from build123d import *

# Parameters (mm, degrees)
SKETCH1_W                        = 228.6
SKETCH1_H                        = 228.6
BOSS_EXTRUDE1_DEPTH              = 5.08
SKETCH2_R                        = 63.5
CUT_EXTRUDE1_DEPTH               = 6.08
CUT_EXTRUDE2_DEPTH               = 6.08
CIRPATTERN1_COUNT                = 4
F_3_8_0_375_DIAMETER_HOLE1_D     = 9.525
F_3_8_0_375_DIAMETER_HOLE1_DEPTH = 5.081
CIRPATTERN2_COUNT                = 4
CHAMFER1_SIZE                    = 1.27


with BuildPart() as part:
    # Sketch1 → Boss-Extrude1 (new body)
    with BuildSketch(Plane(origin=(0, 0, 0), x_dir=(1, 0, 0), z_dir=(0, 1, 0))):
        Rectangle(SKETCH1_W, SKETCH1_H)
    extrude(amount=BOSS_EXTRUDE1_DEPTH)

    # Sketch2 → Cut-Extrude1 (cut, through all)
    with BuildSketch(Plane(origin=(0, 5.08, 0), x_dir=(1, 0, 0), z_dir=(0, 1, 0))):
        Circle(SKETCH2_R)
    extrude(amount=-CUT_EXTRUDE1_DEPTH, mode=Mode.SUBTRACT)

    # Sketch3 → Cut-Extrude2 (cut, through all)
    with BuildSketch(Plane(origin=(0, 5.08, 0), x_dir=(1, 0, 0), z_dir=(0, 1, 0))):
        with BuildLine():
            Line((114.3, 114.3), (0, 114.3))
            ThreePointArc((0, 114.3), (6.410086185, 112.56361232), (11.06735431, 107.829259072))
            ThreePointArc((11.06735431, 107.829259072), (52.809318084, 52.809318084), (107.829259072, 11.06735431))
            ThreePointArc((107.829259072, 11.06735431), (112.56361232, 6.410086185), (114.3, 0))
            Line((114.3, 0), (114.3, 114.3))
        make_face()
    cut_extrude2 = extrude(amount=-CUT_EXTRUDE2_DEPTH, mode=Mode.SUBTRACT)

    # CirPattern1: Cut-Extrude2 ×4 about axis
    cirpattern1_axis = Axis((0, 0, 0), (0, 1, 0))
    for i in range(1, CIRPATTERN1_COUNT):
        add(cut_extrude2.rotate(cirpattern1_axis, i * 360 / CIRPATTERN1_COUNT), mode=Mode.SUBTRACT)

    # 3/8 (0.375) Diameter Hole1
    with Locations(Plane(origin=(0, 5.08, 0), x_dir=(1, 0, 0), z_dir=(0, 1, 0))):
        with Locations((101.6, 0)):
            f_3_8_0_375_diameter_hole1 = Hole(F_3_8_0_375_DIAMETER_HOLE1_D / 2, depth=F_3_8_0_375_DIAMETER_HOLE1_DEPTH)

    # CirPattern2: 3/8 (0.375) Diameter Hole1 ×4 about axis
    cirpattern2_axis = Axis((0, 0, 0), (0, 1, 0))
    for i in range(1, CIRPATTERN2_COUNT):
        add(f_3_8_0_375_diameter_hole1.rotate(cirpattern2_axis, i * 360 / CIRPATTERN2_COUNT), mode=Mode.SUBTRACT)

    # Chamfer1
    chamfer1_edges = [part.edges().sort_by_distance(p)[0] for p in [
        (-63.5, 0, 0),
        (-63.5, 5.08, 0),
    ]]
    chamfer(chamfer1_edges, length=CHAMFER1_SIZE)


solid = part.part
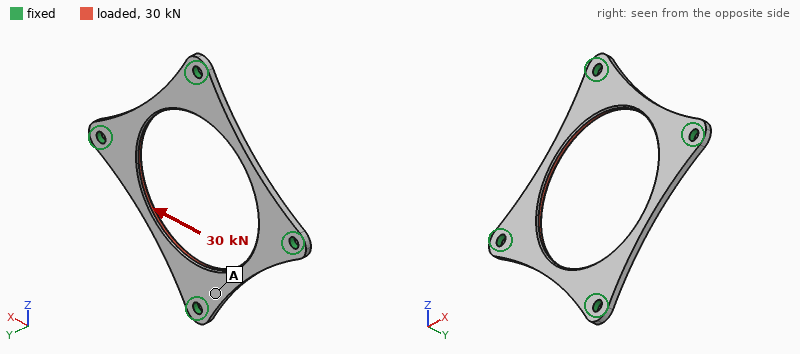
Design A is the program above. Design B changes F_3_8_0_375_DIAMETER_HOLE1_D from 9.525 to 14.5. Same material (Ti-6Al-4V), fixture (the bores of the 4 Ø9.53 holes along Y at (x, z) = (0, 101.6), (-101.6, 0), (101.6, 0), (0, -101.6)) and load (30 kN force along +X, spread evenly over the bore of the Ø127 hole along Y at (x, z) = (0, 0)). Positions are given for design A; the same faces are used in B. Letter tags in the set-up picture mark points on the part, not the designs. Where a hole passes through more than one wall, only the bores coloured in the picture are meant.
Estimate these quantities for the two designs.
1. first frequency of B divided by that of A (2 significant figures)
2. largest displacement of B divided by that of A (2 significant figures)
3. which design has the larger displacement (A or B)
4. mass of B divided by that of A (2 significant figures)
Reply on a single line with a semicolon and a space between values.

1.1; 0.78; A; 0.97
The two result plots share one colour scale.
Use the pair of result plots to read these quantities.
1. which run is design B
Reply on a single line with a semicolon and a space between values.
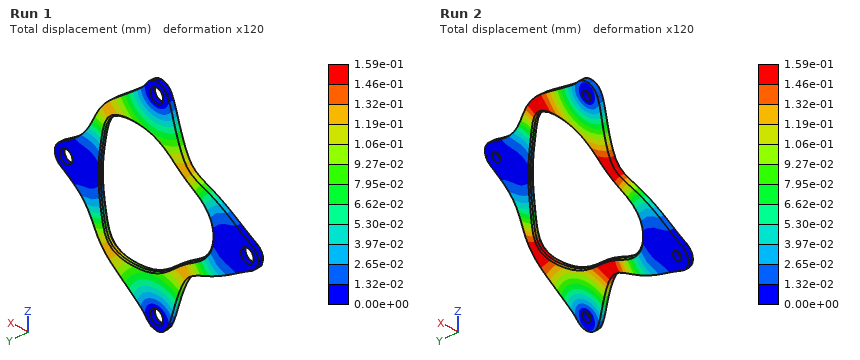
Run 1
